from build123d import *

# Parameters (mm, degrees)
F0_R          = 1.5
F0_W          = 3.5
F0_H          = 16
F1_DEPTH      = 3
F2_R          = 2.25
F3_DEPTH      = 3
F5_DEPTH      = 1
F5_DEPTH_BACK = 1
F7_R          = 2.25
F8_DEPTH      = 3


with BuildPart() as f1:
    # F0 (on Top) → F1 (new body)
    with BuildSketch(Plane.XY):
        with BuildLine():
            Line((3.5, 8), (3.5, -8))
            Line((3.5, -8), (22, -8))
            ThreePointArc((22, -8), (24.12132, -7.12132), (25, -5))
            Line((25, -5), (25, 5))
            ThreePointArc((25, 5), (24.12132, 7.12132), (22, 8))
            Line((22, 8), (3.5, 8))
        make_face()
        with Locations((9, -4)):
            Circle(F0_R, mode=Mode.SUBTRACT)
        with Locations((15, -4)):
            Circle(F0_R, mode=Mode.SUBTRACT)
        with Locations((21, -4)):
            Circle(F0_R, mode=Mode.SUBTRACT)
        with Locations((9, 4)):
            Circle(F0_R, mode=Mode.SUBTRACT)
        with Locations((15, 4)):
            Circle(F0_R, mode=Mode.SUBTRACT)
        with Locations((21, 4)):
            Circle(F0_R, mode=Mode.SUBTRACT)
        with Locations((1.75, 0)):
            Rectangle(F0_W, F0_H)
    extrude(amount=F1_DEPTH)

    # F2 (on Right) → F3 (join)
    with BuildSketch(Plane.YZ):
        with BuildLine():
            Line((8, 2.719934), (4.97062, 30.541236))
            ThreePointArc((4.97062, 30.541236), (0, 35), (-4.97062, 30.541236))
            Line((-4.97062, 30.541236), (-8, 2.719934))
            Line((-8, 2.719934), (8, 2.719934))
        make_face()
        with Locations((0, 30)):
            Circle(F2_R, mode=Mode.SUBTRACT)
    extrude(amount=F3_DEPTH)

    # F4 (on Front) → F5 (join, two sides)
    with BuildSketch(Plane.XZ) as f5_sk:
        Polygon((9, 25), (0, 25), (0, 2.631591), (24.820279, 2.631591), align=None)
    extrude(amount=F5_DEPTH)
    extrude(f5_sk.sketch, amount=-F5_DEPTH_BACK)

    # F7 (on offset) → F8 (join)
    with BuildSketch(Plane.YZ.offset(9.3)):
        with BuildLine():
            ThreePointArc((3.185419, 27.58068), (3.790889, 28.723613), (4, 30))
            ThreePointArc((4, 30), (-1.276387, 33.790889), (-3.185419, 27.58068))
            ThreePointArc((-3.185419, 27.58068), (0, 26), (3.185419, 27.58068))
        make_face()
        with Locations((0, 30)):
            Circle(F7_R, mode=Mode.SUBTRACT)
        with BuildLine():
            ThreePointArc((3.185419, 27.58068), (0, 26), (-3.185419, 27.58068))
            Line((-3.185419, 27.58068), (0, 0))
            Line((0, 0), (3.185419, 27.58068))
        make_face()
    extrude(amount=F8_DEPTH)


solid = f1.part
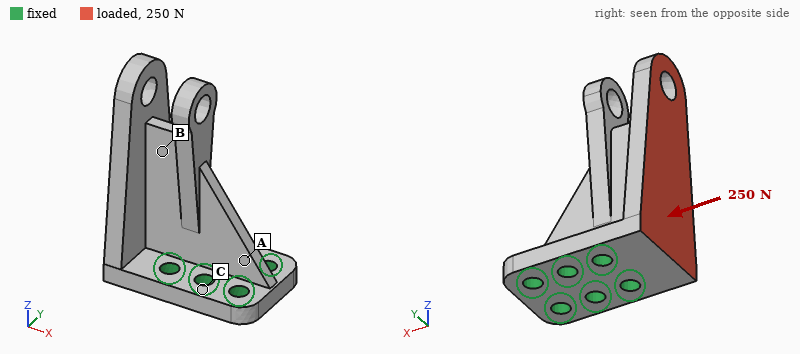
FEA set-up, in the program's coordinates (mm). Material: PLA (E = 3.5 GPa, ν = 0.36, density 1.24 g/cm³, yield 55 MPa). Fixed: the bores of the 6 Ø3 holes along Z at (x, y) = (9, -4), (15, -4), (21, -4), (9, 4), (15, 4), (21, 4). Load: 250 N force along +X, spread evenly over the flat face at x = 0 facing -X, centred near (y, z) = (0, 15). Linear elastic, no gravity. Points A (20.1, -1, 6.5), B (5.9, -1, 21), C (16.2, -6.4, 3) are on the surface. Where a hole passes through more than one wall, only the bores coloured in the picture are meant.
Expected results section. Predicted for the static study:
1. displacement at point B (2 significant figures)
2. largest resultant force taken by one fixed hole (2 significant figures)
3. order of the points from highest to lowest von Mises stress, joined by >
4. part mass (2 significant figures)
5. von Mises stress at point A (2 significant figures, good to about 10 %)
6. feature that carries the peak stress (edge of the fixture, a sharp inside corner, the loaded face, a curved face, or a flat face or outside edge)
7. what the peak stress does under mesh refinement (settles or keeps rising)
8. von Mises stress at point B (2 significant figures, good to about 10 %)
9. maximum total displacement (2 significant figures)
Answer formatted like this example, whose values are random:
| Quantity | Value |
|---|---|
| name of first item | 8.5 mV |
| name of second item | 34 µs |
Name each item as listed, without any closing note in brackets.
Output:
| Quantity | Value |
|---|---|
| displacement at point B | 0.21 mm |
| largest resultant force taken by one fixed hole | 130 N |
| order of the points from highest to lowest von Mises stress, joined by > | A > B > C |
| part mass | 3.8 g |
| von Mises stress at point A | 17 MPa |
| feature that carries the peak stress | edge of the fixture |
| what the peak stress does under mesh refinement | keeps rising |
| von Mises stress at point B | 10 MPa |
| maximum total displacement | 0.55 mm |
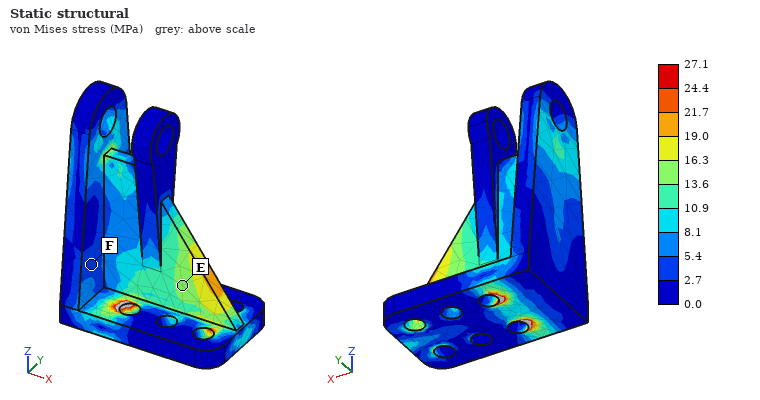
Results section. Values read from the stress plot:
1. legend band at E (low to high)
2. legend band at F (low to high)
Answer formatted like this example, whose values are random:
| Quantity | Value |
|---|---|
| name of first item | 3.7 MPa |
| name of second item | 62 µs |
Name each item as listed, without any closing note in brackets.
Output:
| Quantity | Value |
|---|---|
| legend band at E | 13.6 to 16.3 MPa |
| legend band at F | 2.7 to 5.4 MPa |
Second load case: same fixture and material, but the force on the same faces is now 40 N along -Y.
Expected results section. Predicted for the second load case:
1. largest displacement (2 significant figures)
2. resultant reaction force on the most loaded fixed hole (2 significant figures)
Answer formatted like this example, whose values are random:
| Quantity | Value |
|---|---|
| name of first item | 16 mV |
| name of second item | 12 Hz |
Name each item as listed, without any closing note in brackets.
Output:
| Quantity | Value |
|---|---|
| largest displacement | 0.26 mm |
| resultant reaction force on the most loaded fixed hole | 64 N |
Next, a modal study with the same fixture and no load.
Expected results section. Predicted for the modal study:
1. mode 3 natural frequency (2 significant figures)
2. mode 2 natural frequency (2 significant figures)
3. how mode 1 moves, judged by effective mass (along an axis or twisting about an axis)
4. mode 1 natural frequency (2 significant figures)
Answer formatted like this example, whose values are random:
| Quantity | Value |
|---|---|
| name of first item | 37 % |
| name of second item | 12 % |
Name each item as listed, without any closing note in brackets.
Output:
| Quantity | Value |
|---|---|
| mode 3 natural frequency | 3000 Hz |
| mode 2 natural frequency | 2900 Hz |
| how mode 1 moves, judged by effective mass | along Y |
| mode 1 natural frequency | 1500 Hz |
